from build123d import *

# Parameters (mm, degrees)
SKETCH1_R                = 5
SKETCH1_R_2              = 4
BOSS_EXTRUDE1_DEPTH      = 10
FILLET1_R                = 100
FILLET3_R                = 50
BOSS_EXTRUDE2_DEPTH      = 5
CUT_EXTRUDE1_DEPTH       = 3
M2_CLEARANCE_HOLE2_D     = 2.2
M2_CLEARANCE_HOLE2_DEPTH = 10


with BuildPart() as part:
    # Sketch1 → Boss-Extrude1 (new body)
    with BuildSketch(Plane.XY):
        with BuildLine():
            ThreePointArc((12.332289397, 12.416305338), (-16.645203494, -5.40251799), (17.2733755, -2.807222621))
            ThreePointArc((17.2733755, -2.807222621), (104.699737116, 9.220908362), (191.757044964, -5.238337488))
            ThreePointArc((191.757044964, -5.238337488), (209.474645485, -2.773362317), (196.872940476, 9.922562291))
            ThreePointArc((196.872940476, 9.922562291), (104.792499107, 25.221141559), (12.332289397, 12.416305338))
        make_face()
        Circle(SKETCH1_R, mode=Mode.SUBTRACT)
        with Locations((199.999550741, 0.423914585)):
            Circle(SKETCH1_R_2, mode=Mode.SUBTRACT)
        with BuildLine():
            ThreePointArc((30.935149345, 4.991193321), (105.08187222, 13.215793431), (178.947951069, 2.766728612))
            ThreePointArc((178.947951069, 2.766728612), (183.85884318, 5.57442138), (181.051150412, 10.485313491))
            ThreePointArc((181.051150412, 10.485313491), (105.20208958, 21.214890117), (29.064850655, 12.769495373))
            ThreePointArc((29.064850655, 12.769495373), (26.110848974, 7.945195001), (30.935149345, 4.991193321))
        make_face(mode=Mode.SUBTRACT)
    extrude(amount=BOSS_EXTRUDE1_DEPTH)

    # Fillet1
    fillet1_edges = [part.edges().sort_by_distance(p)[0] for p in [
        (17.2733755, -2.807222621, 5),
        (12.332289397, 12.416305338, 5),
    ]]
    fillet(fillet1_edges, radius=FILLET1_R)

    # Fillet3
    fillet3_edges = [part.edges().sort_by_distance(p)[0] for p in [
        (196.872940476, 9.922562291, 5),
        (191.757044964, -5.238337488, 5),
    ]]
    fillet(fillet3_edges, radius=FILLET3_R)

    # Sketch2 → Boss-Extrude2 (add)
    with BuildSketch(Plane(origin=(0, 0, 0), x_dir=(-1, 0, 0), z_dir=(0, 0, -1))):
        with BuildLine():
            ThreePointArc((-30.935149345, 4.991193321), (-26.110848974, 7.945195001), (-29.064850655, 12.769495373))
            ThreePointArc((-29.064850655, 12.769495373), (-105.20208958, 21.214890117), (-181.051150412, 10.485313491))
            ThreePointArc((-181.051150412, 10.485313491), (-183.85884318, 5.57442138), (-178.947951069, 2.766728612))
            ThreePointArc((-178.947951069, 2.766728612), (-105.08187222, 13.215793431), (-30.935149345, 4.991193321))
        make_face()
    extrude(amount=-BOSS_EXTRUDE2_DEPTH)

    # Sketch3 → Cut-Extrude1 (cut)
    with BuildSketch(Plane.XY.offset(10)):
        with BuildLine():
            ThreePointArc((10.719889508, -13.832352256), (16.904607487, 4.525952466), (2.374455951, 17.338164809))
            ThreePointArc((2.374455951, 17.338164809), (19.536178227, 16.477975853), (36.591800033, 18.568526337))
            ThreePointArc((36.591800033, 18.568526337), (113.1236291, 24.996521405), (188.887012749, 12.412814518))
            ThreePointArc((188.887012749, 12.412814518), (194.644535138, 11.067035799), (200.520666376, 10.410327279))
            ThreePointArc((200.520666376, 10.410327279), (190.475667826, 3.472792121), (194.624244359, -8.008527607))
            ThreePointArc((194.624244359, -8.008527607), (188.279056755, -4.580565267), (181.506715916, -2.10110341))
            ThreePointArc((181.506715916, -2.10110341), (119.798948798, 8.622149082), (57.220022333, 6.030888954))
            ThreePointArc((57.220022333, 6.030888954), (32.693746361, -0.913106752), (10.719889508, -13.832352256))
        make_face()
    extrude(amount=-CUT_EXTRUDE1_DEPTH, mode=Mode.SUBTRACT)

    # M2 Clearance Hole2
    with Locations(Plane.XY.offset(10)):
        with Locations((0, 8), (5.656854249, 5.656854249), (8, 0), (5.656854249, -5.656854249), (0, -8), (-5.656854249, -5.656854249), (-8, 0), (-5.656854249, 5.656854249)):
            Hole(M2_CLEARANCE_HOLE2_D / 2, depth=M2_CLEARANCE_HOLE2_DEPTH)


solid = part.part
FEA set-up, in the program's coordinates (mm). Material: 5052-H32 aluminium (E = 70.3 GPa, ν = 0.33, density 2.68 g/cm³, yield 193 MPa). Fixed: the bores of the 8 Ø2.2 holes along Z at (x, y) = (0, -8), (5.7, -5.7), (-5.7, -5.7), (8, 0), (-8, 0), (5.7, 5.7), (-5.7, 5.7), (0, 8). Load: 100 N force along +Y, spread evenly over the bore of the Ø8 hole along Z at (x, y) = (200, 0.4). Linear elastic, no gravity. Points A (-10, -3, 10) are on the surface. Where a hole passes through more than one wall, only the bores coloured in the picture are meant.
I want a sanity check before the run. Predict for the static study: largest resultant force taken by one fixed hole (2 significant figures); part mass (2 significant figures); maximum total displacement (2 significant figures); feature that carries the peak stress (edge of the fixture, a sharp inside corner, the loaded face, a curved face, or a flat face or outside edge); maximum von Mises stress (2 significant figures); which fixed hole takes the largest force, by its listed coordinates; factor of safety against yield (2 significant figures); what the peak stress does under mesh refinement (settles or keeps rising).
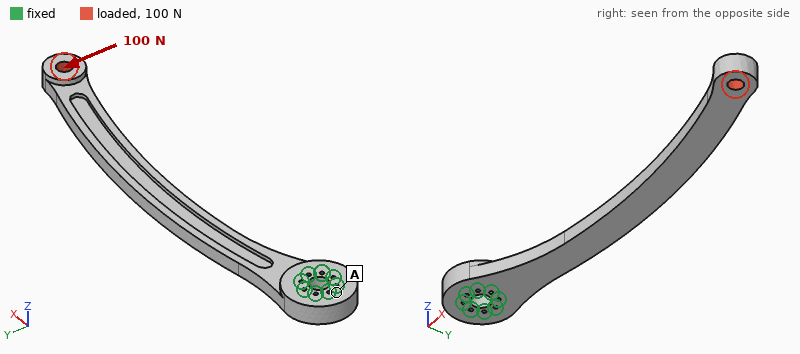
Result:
610 N
79 g
1.3 mm
a curved face
54 MPa
(5.7, -5.7)
3.6
settles
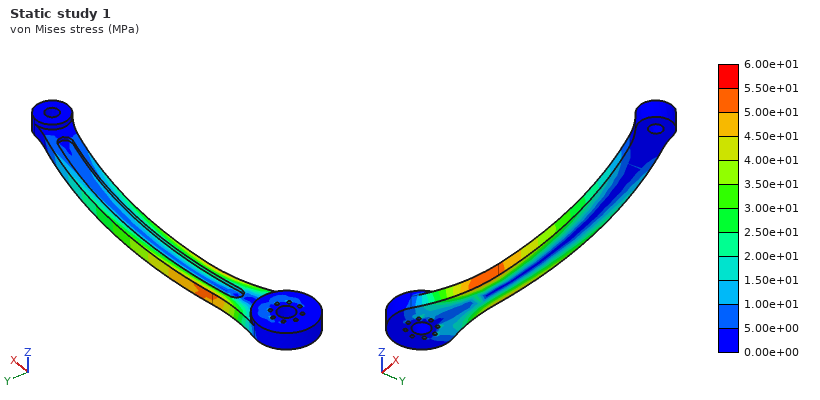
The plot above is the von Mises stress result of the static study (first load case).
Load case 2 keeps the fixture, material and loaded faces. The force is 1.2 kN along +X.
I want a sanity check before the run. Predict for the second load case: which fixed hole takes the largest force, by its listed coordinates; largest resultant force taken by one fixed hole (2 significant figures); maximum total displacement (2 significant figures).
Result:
(8, 0)
400 N
2.4 mm
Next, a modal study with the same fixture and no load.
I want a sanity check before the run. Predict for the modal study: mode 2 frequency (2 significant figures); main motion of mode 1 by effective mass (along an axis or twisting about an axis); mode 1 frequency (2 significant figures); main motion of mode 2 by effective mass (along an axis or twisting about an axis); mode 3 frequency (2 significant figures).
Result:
360 Hz
along Z
130 Hz
along Y
790 Hz
